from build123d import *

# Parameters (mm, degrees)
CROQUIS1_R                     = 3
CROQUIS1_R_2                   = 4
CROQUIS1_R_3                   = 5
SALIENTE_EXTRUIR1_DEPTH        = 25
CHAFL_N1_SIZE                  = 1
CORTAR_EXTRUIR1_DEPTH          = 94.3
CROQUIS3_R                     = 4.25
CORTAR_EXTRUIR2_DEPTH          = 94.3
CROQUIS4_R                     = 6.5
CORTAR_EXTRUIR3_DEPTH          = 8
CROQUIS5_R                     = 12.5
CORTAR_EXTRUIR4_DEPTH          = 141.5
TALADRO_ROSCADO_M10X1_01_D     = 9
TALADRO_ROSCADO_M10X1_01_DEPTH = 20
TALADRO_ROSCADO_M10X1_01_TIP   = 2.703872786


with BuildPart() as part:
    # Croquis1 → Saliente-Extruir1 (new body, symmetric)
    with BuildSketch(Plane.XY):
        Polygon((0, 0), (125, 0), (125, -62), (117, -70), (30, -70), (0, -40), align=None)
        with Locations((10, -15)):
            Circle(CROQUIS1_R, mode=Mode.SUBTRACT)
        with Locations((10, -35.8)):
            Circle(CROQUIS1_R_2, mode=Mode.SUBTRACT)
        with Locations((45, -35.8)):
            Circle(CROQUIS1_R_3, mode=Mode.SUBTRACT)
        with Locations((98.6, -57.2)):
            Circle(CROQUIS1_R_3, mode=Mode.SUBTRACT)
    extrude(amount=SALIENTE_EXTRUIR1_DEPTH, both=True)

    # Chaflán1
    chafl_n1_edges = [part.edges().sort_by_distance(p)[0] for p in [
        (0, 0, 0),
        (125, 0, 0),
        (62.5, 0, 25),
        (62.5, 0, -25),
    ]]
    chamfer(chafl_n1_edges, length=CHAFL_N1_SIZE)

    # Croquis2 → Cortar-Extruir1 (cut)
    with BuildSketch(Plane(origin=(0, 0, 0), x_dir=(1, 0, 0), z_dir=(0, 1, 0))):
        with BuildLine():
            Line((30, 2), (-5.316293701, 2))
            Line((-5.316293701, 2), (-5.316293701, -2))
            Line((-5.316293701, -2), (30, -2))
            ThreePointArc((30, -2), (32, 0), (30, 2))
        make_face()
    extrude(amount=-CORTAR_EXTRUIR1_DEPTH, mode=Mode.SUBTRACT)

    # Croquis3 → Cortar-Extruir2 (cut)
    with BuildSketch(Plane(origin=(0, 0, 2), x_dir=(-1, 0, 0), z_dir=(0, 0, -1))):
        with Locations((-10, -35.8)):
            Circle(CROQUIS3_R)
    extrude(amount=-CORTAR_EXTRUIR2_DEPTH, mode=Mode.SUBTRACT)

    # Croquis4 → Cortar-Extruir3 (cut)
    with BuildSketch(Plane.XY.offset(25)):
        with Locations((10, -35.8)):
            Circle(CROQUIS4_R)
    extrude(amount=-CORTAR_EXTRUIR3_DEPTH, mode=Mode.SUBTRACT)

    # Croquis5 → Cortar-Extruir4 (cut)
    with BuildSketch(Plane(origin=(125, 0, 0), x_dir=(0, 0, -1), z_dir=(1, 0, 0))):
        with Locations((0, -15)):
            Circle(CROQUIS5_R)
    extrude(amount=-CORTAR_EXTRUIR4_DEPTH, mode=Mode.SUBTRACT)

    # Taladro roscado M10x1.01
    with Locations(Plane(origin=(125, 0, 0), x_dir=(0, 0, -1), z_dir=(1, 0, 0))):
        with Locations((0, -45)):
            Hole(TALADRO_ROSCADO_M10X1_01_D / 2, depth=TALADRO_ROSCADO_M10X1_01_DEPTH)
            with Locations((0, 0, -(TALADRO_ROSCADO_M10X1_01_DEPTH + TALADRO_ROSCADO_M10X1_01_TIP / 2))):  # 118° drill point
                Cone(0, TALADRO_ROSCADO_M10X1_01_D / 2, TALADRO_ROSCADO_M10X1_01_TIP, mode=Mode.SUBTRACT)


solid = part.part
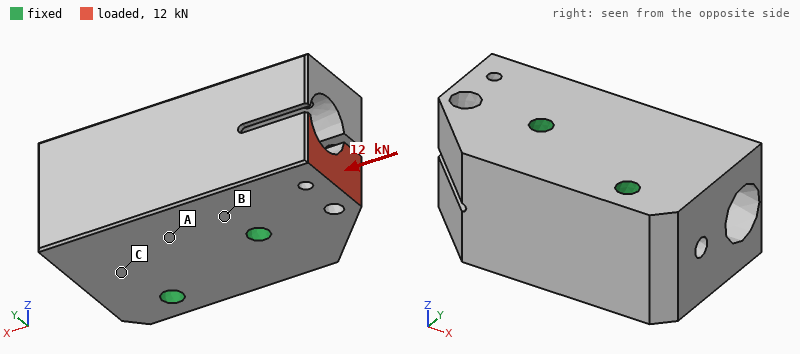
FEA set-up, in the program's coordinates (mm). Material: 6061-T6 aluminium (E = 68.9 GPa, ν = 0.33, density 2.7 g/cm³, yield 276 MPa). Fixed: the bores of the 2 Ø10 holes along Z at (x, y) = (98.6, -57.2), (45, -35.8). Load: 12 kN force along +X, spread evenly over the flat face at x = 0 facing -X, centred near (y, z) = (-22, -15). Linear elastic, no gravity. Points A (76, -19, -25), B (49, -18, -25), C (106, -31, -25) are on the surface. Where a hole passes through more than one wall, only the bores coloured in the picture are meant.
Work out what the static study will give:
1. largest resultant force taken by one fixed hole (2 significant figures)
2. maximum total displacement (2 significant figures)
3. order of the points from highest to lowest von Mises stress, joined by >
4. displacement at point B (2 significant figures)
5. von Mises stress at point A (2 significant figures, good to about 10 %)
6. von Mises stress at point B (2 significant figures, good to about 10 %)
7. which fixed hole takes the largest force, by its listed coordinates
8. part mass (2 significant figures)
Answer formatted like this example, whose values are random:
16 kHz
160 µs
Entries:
11 kN
25 µm
B > A > C
5.5 µm
6.7 MPa
14 MPa
(45, -35.8)
900 g
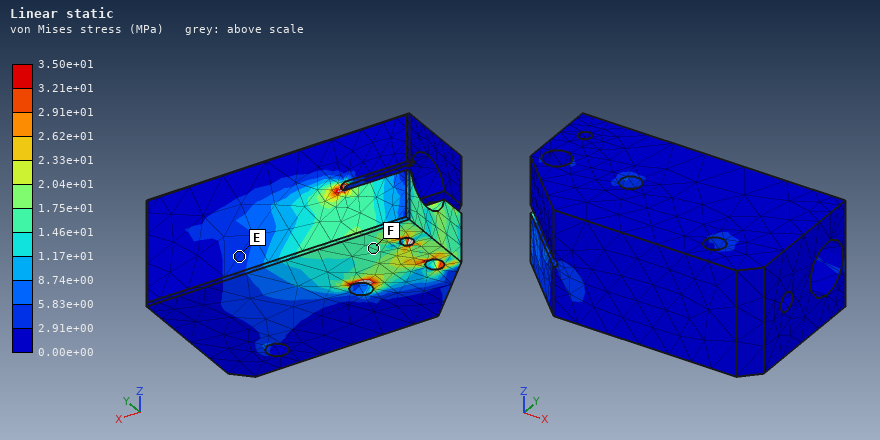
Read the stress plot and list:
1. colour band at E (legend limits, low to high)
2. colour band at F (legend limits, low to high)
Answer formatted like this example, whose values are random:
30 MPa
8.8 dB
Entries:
2.91e+00 to 5.83e+00 MPa
1.46e+01 to 1.75e+01 MPa
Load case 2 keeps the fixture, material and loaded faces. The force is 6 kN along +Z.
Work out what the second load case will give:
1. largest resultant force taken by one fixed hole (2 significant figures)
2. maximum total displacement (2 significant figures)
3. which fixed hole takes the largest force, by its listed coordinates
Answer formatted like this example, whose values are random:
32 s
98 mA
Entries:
7.0 kN
96 µm
(45, -35.8)
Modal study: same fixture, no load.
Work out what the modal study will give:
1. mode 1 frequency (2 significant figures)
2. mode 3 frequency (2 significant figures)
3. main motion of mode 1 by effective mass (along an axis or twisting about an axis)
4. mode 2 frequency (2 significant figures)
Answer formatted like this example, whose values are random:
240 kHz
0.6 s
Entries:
8100 Hz
9200 Hz
along Z
8900 Hz
